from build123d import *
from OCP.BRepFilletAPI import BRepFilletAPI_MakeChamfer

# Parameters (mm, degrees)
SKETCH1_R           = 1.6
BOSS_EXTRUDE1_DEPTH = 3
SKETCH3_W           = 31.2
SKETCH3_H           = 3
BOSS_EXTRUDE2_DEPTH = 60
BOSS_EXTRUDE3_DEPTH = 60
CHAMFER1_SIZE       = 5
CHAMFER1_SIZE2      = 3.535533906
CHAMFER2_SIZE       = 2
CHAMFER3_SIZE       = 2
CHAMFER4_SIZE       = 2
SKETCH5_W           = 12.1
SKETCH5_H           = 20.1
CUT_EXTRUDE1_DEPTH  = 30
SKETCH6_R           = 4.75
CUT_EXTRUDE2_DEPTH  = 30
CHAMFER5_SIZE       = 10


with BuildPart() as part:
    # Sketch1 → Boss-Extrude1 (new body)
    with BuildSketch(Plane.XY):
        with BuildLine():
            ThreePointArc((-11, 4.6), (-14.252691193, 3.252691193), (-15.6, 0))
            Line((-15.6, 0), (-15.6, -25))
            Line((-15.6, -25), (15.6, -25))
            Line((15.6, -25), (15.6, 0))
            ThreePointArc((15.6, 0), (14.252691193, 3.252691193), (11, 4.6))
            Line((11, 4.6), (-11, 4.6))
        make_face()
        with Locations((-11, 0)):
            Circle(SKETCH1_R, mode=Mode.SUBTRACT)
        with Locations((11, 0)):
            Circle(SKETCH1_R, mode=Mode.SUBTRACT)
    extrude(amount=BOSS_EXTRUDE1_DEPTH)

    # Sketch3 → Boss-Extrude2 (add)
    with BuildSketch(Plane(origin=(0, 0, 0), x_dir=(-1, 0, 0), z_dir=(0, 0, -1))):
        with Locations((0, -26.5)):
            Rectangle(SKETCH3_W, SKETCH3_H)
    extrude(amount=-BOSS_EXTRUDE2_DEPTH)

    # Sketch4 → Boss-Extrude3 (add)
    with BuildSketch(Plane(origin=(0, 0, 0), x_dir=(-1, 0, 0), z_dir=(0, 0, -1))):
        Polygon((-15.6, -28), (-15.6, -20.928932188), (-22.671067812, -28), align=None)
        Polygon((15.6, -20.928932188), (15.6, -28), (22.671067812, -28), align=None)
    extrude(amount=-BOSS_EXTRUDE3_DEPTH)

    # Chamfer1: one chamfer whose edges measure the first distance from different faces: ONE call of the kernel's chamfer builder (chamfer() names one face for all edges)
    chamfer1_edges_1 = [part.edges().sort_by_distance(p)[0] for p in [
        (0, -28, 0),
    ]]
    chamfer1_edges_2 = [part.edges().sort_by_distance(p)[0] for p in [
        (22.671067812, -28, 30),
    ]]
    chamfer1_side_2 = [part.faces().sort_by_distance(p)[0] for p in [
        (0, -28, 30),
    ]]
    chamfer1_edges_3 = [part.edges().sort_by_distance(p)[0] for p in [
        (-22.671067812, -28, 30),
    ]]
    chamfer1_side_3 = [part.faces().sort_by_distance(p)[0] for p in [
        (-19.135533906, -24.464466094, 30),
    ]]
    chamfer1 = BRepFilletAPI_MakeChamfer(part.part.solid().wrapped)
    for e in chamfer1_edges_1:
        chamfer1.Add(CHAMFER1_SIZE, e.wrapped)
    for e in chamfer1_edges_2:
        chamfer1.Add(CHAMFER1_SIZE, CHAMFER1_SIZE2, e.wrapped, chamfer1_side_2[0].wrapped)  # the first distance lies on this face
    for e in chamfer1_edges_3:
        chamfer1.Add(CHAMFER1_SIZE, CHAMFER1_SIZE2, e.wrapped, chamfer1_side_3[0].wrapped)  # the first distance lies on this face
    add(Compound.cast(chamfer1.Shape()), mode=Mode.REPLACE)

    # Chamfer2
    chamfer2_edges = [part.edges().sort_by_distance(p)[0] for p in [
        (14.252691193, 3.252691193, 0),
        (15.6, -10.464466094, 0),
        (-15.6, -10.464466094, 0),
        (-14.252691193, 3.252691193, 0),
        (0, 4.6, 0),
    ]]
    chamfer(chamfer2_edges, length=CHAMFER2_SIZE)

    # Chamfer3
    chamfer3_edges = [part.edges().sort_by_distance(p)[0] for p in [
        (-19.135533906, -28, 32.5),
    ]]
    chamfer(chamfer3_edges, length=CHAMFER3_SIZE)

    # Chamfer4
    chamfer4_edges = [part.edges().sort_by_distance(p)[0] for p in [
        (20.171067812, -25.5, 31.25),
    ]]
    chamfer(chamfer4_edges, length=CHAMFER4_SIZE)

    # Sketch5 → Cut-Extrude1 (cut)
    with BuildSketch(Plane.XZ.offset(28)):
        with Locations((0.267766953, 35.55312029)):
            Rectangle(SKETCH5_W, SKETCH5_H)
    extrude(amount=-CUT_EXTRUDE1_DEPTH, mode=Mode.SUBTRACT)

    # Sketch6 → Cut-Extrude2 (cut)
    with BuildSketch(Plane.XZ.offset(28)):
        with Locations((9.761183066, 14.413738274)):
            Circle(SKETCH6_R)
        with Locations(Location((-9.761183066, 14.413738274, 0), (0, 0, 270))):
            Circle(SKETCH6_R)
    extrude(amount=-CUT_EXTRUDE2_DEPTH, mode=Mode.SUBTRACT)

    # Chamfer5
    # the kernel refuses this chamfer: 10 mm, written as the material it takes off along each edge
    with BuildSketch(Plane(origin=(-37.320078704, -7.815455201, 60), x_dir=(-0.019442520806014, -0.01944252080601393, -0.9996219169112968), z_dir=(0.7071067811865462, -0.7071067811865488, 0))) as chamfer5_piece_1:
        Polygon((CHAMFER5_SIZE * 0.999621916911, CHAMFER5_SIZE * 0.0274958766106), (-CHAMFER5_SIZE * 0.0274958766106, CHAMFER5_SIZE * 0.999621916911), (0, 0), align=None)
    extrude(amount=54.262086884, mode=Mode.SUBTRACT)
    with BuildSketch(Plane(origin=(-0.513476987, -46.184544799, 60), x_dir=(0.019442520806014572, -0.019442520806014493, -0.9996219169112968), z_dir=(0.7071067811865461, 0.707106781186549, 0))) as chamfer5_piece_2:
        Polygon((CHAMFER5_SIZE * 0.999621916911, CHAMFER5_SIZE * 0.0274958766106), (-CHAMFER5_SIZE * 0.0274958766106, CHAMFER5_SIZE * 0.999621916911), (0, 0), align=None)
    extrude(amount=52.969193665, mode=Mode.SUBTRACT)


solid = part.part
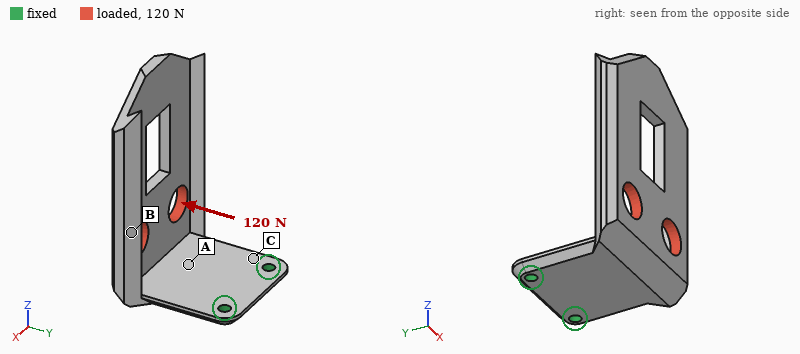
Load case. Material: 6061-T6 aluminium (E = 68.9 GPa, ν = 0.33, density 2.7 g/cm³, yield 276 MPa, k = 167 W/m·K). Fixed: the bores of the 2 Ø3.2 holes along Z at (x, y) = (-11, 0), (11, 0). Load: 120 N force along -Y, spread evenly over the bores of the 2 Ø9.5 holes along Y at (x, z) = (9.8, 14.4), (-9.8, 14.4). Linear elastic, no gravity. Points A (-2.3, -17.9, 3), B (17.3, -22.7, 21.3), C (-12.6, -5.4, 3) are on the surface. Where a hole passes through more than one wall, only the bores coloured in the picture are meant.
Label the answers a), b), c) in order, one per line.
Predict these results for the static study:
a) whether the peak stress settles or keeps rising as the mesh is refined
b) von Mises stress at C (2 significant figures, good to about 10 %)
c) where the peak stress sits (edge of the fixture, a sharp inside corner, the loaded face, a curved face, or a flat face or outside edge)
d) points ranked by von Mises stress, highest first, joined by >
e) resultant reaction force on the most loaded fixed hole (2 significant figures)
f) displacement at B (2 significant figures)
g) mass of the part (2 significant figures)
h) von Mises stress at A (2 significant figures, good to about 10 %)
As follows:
a) keeps rising
b) 41 MPa
c) a sharp inside corner
d) C > A > B
e) 60 N
f) 0.26 mm
g) 22 g
h) 29 MPa
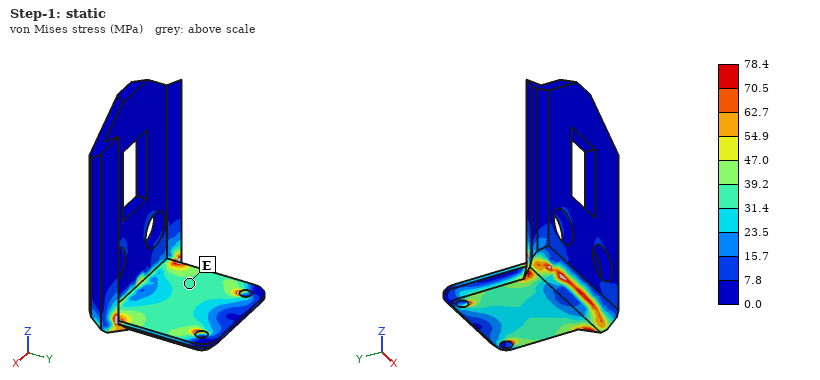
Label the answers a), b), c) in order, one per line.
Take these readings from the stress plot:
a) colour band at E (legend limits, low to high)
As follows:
a) 31.4 to 39.2 MPa
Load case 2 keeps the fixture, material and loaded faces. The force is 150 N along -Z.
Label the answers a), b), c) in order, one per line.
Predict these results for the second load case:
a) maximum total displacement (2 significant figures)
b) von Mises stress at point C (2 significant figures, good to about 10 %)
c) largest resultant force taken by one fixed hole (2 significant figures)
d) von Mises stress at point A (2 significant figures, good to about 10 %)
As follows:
a) 0.79 mm
b) 81 MPa
c) 75 N
d) 27 MPa
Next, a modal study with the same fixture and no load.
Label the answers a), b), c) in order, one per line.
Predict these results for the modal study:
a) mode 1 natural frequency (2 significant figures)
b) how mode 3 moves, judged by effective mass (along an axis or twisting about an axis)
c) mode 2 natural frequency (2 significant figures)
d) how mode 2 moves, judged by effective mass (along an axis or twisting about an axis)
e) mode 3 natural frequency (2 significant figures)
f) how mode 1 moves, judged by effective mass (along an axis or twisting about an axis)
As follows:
a) 400 Hz
b) along Z
c) 760 Hz
d) along X
e) 1600 Hz
f) along Y
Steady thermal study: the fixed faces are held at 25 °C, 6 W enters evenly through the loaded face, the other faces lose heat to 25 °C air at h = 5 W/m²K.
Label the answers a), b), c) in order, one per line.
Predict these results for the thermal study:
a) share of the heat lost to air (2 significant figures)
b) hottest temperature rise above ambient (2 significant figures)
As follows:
a) 6.4 %
b) 16 K
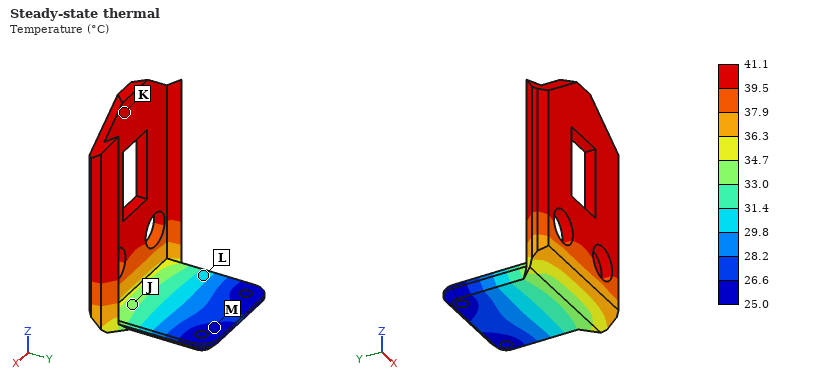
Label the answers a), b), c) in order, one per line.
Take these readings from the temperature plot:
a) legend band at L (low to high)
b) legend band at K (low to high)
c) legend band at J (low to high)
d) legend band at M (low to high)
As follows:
a) 29.8 to 31.4 °C
b) 39.5 to 41.1 °C
c) 33.0 to 34.7 °C
d) 25.0 to 26.6 °C
